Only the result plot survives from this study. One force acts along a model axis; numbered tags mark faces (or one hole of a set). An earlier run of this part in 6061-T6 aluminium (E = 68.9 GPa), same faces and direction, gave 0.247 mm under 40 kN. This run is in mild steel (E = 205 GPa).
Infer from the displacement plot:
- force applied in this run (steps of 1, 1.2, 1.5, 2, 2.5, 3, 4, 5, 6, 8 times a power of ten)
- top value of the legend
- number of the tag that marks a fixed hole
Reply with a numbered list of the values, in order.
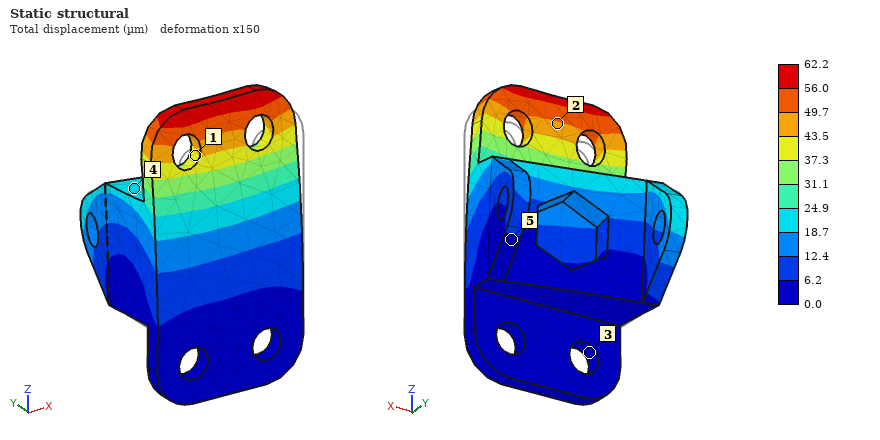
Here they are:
1. 30 kN
2. 62.2 µm
3. 3
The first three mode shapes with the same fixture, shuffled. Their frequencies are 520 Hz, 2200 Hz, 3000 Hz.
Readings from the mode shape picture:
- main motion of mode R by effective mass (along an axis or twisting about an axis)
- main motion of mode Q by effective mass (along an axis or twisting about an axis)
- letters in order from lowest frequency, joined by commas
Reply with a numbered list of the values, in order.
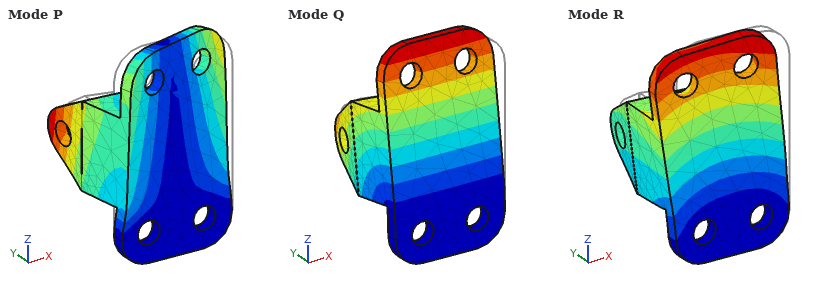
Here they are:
1. along X
2. along Y
3. Q, P, R
